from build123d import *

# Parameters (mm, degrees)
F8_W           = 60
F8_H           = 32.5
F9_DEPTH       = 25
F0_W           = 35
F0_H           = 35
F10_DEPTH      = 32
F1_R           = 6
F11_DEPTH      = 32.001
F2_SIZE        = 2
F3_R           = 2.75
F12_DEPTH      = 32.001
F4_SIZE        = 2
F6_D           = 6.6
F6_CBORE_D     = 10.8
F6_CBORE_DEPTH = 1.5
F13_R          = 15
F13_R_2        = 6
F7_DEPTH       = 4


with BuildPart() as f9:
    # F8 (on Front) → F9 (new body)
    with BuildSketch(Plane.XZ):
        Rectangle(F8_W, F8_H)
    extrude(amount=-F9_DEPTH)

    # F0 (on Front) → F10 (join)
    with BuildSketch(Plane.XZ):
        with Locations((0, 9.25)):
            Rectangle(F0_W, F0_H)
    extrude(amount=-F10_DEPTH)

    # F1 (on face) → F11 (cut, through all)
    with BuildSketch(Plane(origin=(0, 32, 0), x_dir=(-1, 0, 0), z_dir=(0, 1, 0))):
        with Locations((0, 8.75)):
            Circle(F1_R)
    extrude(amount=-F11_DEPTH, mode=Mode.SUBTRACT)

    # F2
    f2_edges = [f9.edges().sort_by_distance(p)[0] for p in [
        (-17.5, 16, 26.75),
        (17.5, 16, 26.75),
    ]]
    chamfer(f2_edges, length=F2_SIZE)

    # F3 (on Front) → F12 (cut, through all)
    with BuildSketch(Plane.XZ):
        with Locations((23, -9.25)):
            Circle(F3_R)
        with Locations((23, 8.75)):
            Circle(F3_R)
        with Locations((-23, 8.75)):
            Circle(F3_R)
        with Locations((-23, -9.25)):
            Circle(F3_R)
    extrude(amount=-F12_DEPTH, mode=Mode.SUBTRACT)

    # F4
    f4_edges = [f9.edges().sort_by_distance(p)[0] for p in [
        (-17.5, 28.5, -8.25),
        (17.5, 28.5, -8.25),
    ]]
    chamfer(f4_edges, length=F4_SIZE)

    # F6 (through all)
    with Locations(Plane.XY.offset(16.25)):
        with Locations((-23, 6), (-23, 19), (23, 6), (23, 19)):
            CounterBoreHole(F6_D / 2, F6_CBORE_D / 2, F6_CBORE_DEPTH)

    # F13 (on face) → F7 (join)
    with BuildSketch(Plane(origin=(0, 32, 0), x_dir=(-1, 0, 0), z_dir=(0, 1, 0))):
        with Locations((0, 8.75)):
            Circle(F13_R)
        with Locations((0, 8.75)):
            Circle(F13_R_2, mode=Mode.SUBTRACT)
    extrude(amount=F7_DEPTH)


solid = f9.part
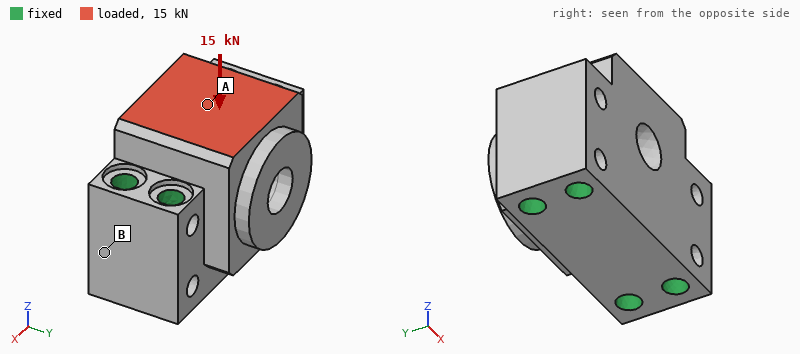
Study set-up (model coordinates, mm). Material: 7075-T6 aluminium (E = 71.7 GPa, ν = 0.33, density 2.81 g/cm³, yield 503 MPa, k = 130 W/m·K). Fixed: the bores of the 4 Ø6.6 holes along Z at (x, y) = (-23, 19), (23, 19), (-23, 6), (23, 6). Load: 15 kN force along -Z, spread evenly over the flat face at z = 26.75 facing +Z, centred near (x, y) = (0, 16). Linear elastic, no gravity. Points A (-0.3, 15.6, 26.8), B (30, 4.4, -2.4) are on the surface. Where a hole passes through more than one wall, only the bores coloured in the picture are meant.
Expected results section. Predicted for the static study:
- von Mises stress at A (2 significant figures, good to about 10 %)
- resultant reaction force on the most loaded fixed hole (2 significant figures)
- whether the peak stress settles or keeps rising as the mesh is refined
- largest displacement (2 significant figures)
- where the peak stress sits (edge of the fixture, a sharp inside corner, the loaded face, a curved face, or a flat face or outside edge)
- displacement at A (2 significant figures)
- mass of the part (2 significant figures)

14 MPa
4.8 kN
keeps rising
11 µm
edge of the fixture
9.5 µm
170 g
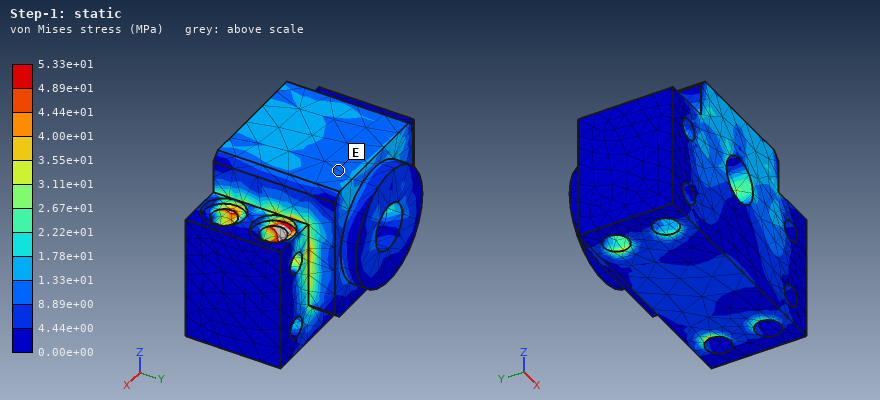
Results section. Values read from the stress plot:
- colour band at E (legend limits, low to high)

8.89e+00 to 1.33e+01 MPa
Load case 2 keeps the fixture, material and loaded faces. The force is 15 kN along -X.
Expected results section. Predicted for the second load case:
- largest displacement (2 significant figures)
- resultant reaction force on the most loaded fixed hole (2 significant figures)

18 µm
5.6 kN
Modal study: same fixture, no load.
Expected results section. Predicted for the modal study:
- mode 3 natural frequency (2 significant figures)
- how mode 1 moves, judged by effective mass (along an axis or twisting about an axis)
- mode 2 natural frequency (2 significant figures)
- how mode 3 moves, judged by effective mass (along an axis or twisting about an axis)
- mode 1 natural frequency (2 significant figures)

31 kHz
along Y
27 kHz
along X
17 kHz
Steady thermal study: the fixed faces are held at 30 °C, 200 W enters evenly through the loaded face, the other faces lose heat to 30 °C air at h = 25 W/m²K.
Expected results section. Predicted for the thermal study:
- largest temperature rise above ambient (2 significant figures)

39 K
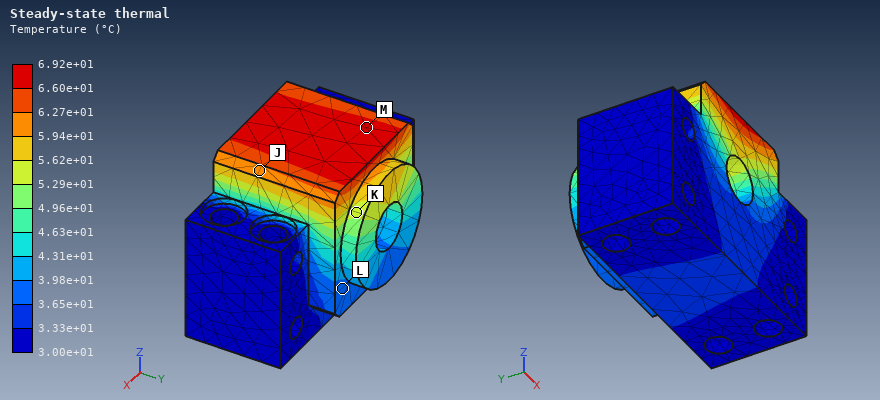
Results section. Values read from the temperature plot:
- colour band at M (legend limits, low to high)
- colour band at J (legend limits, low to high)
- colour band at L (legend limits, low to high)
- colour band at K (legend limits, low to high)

6.60e+01 to 6.92e+01 °C
5.94e+01 to 6.27e+01 °C
3.65e+01 to 3.98e+01 °C
5.29e+01 to 5.62e+01 °C
